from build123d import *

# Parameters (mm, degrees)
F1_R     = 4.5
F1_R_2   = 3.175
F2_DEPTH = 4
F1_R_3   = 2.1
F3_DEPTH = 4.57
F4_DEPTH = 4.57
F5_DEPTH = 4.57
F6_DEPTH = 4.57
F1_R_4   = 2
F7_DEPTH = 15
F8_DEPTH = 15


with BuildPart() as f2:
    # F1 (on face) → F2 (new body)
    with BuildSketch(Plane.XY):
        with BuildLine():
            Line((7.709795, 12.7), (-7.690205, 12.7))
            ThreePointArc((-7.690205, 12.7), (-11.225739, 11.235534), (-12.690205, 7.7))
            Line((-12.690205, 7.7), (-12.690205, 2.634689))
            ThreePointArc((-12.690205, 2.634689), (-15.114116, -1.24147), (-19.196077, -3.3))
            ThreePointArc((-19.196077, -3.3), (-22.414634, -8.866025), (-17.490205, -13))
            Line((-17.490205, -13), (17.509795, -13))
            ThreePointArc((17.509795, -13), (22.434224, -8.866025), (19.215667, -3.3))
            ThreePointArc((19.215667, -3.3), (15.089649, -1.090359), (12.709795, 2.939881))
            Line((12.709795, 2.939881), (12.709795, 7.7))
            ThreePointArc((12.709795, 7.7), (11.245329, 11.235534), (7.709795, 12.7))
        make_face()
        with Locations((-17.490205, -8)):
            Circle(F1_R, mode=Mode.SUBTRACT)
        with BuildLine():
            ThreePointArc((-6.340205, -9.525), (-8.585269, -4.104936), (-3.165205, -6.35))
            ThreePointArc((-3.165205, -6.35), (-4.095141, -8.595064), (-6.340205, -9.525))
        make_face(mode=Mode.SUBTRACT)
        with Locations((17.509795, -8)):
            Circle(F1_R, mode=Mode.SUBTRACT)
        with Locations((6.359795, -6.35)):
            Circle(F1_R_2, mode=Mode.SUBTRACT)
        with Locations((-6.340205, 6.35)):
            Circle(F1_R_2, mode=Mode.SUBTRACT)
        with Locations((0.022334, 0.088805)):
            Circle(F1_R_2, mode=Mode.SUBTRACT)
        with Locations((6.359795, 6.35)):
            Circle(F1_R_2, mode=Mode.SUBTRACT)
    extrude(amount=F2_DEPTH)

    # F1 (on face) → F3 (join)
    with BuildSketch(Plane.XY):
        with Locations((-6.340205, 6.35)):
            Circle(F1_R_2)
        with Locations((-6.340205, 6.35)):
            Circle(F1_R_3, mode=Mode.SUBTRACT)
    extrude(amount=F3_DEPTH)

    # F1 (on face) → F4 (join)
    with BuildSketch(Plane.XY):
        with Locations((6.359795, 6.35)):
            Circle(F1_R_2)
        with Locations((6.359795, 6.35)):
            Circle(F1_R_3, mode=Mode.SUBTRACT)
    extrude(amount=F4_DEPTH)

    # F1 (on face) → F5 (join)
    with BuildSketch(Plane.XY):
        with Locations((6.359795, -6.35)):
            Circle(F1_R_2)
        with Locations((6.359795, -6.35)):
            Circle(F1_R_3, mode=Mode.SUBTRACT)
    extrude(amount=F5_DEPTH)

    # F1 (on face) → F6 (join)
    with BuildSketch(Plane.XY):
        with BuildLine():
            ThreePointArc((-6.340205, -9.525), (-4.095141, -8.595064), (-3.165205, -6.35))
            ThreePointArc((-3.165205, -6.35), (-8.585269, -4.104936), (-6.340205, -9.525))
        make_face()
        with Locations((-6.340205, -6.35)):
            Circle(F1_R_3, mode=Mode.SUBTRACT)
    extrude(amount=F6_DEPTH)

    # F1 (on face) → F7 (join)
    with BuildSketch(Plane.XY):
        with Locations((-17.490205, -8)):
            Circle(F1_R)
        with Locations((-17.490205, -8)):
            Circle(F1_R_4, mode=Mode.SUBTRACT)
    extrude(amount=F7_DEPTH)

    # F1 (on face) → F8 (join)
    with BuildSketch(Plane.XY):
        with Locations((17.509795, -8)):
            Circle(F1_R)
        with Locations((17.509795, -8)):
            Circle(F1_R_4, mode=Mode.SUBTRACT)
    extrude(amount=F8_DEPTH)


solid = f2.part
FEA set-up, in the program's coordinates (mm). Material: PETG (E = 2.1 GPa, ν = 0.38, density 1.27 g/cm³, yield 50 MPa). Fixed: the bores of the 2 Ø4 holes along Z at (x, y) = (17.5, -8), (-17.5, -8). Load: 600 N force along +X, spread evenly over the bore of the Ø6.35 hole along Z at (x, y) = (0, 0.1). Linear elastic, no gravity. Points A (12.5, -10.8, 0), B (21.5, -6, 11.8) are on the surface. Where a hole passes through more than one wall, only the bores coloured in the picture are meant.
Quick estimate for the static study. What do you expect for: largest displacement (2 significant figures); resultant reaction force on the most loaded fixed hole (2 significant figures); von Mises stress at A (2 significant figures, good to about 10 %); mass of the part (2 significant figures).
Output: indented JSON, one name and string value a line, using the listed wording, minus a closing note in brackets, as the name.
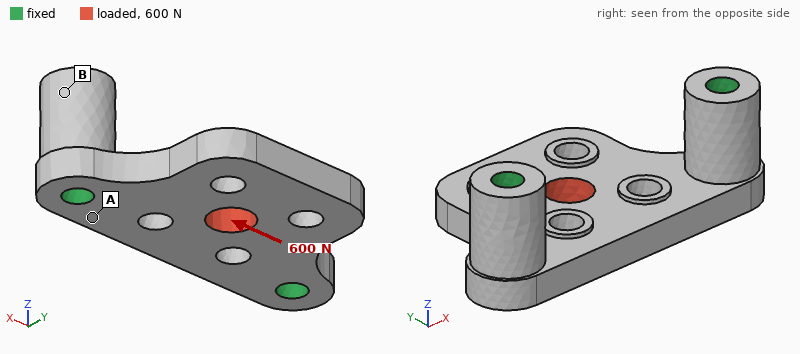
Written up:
{
  "largest displacement": "0.10 mm",
  "resultant reaction force on the most loaded fixed hole": "330 N",
  "von Mises stress at A": "3.0 MPa",
  "mass of the part": "5.2 g"
}
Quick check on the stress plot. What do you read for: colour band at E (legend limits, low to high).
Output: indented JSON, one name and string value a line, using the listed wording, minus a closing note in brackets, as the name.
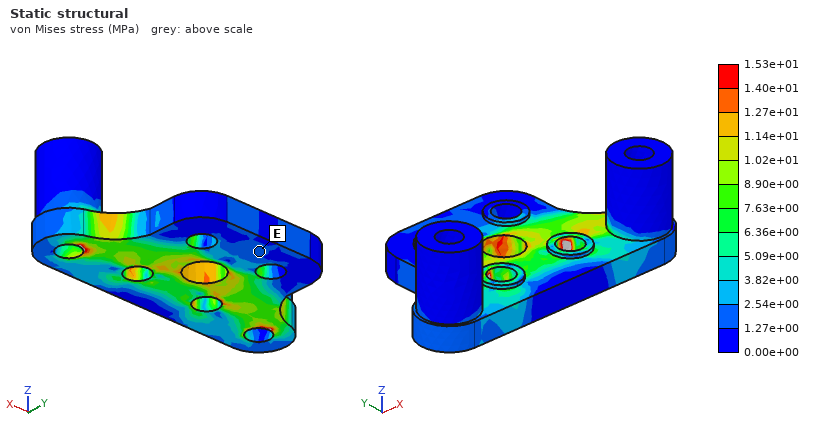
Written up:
{
  "colour band at E": "1.27e+00 to 2.54e+00 MPa"
}
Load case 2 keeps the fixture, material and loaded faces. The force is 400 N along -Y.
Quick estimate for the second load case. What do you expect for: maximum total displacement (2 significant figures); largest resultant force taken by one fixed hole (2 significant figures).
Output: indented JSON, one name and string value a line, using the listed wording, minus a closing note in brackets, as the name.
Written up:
{
  "maximum total displacement": "0.11 mm",
  "largest resultant force taken by one fixed hole": "220 N"
}
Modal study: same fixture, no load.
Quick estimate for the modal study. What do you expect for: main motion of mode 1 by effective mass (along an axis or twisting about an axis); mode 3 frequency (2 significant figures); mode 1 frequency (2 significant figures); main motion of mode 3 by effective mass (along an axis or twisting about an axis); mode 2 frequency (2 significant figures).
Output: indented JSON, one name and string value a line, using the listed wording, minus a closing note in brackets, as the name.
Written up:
{
  "main motion of mode 1 by effective mass": "along Z",
  "mode 3 frequency": "5300 Hz",
  "mode 1 frequency": "1700 Hz",
  "main motion of mode 3 by effective mass": "along Z",
  "mode 2 frequency": "4300 Hz"
}
